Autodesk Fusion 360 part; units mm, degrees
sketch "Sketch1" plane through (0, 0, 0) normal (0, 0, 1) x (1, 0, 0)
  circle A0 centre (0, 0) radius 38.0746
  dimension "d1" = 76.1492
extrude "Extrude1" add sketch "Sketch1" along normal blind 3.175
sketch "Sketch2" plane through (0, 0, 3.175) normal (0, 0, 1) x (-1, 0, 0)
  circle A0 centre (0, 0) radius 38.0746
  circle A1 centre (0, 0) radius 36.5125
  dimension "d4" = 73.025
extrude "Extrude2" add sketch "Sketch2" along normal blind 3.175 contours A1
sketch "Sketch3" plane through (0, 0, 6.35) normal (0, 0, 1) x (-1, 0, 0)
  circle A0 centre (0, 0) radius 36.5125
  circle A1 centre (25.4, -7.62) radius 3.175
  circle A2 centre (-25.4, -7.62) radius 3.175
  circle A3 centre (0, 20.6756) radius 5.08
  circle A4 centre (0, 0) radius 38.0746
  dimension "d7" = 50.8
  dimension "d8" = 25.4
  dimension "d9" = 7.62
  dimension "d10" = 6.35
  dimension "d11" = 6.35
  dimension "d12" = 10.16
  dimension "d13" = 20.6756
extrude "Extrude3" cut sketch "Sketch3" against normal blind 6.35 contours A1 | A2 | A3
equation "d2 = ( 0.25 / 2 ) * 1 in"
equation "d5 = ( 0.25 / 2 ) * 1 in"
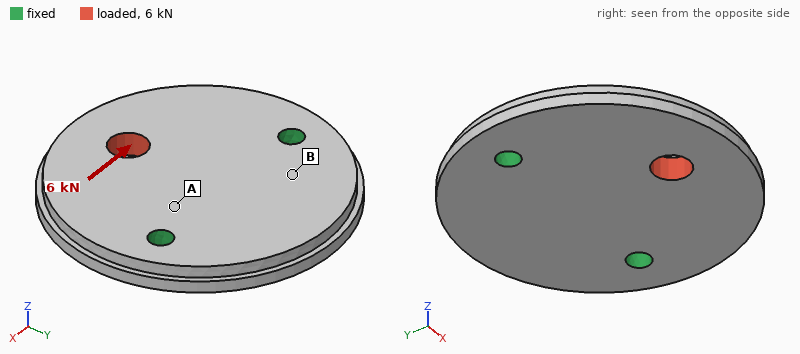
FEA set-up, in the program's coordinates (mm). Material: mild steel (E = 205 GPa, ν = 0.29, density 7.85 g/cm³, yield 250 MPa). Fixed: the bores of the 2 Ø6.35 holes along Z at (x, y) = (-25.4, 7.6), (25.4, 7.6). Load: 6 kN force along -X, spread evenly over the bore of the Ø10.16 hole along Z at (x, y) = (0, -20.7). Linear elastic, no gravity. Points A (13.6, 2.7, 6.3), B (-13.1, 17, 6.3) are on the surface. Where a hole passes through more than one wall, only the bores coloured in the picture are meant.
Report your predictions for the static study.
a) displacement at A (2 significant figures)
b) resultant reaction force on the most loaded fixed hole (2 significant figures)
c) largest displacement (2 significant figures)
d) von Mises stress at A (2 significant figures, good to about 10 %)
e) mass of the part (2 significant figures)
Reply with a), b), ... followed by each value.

a) 1.5 µm
b) 4.3 kN
c) 9.9 µm
d) 26 MPa
e) 210 g
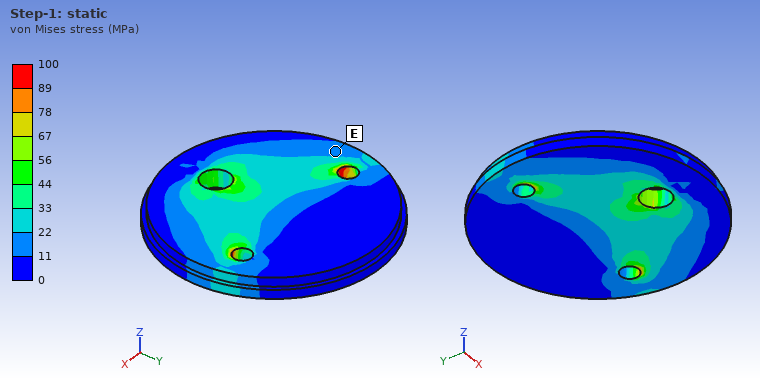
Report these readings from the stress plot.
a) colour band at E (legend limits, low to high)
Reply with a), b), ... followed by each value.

a) 11 to 22 MPa
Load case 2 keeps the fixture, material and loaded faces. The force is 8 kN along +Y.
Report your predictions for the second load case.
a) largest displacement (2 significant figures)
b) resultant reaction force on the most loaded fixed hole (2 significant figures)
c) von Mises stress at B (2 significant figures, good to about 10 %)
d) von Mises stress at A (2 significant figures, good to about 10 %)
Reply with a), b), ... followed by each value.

a) 8.0 µm
b) 4.1 kN
c) 12 MPa
d) 23 MPa
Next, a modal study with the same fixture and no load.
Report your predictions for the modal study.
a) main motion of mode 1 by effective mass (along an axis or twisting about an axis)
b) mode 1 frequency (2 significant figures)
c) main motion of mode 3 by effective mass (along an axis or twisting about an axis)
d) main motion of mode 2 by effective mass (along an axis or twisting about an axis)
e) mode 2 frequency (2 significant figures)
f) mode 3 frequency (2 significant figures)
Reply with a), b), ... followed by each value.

a) along Z
b) 3000 Hz
c) twisting about Y
d) along Z
e) 6200 Hz
f) 7000 Hz
